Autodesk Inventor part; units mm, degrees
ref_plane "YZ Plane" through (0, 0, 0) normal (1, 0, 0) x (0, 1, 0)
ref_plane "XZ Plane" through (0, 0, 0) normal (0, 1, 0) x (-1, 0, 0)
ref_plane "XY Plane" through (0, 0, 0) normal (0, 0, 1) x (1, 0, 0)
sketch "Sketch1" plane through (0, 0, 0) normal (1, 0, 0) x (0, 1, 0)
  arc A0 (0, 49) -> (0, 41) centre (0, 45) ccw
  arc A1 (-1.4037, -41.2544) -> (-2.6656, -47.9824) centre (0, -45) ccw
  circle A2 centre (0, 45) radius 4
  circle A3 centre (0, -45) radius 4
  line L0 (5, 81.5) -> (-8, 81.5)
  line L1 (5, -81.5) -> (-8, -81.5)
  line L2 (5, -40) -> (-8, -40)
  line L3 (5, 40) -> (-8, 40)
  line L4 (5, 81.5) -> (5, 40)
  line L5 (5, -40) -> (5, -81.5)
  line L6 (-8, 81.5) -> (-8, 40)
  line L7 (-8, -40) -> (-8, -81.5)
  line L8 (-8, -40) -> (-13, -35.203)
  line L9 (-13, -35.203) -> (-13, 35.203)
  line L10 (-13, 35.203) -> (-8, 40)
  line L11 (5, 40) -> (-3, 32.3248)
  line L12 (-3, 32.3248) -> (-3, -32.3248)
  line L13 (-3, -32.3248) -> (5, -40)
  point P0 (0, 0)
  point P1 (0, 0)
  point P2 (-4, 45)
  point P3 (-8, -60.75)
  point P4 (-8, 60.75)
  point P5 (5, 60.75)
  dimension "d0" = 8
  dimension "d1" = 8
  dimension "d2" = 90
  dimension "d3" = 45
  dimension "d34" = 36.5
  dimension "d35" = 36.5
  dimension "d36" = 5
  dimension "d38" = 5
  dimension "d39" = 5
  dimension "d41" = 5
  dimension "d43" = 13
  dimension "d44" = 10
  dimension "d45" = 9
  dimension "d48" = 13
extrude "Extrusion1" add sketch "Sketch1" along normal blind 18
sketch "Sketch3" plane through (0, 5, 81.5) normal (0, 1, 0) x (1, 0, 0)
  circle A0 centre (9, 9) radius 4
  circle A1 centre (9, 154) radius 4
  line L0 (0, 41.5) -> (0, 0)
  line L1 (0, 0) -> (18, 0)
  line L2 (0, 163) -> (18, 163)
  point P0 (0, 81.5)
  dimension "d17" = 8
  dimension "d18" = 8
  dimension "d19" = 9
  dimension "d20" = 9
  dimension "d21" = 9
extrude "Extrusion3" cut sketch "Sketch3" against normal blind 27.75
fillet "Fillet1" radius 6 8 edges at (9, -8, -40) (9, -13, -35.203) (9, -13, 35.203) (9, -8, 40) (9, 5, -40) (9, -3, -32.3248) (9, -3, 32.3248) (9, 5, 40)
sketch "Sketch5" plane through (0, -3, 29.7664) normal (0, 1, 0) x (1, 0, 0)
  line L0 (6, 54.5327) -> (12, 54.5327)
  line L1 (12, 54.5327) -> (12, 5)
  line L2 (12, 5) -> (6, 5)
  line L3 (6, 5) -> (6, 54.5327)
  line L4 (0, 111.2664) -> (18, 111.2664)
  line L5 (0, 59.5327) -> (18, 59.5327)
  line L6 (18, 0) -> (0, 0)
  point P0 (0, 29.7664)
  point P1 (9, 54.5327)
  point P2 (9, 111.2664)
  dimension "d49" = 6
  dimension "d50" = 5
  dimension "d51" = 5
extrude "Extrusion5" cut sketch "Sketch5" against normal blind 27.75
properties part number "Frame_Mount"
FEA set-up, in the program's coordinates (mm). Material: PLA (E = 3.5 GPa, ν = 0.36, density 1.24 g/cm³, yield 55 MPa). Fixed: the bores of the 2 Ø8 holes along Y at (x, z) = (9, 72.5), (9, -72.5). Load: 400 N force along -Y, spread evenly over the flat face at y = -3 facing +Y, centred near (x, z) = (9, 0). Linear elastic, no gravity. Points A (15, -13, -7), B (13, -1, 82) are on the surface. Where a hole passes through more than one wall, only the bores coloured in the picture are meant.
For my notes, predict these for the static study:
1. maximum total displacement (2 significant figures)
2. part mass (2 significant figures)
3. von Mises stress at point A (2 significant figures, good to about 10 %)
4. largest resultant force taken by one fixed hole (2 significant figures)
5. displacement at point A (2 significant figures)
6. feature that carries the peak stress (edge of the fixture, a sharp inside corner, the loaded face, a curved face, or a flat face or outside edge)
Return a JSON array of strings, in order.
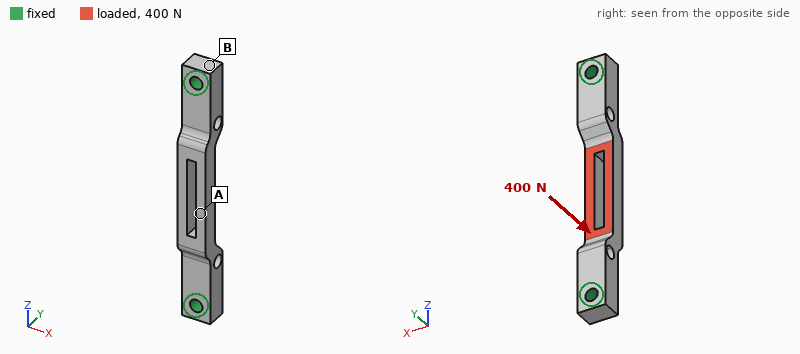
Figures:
["0.61 mm", "35 g", "15 MPa", "470 N", "0.59 mm", "a curved face"]
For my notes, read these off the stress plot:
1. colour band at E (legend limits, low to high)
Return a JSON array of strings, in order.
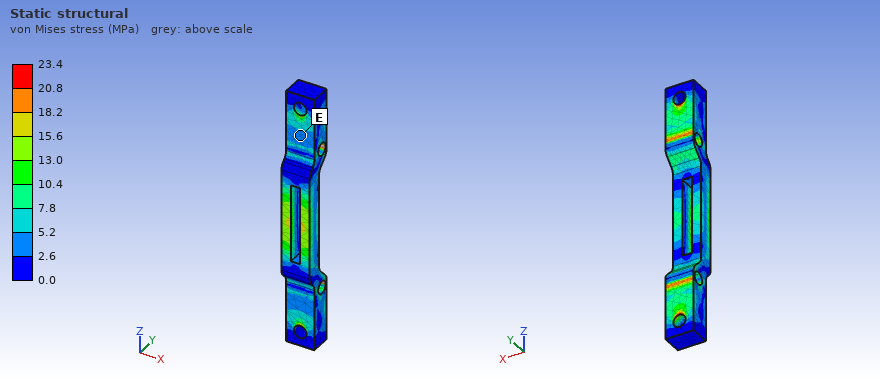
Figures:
["2.6 to 5.2 MPa"]
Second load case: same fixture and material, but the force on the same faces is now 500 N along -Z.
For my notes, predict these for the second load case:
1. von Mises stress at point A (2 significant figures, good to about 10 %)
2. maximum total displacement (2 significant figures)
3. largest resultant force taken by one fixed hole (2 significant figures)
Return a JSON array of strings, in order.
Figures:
["0.63 MPa", "65 µm", "250 N"]
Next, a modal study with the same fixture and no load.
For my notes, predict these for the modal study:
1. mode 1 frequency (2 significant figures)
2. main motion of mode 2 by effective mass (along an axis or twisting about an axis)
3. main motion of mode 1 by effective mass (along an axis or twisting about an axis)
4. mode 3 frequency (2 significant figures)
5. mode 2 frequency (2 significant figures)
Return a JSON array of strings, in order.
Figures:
["1300 Hz", "along X", "along Y", "2100 Hz", "1400 Hz"]
